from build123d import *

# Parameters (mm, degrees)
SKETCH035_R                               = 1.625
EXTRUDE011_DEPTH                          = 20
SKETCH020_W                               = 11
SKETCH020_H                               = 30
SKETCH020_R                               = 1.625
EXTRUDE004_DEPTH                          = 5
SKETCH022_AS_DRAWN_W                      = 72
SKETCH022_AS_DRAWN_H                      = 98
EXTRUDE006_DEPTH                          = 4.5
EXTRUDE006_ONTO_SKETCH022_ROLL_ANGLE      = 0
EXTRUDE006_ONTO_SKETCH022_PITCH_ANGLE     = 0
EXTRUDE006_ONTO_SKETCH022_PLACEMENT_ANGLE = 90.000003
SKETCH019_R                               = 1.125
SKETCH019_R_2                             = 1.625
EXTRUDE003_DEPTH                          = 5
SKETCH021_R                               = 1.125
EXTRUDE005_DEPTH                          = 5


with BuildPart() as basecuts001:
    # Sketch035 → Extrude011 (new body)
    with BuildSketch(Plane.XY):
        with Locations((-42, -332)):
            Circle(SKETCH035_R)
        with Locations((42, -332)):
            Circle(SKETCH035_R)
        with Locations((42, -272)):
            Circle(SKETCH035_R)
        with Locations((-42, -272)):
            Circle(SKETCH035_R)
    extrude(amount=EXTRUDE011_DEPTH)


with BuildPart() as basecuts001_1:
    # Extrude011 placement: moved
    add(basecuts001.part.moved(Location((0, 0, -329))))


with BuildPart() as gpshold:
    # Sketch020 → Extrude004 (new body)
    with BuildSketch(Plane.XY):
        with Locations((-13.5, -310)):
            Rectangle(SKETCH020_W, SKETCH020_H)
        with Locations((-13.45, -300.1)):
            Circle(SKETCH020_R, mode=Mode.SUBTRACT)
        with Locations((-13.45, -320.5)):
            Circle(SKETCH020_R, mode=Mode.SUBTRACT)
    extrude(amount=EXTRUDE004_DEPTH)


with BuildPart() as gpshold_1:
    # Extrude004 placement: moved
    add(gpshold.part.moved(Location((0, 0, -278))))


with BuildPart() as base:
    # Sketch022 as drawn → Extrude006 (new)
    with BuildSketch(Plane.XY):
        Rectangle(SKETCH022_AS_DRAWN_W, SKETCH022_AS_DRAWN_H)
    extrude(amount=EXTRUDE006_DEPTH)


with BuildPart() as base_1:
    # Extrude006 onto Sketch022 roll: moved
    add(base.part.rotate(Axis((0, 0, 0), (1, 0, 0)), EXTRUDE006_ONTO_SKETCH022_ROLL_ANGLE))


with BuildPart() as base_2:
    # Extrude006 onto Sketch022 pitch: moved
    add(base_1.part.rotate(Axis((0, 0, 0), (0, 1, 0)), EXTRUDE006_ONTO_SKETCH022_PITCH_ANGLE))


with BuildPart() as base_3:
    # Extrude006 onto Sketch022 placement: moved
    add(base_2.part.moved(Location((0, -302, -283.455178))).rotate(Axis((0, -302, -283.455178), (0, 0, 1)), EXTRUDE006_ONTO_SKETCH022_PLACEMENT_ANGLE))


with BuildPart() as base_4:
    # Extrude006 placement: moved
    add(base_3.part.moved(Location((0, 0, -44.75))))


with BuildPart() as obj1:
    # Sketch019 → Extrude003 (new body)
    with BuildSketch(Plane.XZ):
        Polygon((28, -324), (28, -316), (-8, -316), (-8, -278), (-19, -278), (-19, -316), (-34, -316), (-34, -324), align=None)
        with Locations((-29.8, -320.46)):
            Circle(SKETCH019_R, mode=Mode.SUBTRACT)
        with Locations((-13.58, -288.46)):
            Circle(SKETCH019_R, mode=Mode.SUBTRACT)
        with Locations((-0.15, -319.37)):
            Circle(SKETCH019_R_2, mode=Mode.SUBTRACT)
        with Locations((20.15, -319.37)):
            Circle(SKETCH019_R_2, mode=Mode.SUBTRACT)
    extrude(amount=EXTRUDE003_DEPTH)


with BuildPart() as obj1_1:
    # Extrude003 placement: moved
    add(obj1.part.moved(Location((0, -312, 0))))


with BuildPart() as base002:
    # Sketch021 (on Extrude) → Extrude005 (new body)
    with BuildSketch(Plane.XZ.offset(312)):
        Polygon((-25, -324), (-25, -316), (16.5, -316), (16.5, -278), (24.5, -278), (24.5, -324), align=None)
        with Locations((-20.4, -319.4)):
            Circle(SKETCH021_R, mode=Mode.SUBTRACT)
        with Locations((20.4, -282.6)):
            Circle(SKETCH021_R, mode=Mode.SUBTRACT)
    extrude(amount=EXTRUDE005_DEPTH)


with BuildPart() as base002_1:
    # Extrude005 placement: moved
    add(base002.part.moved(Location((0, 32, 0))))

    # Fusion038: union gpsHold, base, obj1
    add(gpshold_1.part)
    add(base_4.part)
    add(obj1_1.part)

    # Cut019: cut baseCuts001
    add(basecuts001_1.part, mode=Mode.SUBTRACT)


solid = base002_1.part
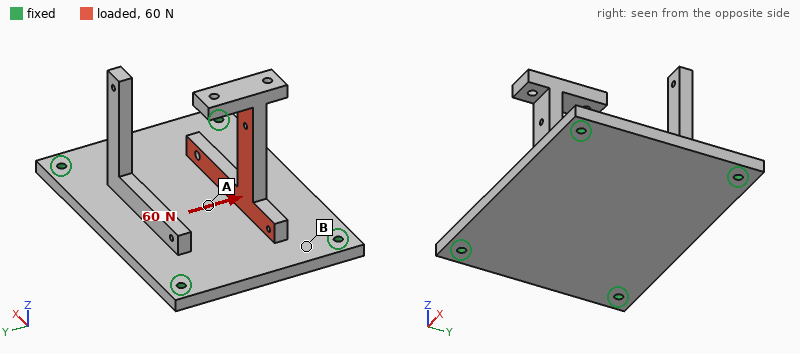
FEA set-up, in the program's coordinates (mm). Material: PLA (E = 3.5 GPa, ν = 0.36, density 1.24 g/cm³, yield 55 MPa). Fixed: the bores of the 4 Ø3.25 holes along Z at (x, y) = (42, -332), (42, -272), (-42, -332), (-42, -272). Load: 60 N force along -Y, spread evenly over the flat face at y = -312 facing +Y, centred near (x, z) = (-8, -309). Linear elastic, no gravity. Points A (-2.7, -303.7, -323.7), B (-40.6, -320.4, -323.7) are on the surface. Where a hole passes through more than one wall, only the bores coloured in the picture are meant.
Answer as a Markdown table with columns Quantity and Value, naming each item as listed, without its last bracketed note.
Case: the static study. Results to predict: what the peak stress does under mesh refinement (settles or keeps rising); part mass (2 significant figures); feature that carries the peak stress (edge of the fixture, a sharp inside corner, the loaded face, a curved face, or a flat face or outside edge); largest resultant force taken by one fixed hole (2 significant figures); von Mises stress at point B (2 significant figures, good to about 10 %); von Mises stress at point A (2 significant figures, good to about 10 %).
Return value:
| Quantity | Value |
|---|---|
| what the peak stress does under mesh refinement | keeps rising |
| part mass | 51 g |
| feature that carries the peak stress | a sharp inside corner |
| largest resultant force taken by one fixed hole | 25 N |
| von Mises stress at point B | 0.98 MPa |
| von Mises stress at point A | 1.9 MPa |
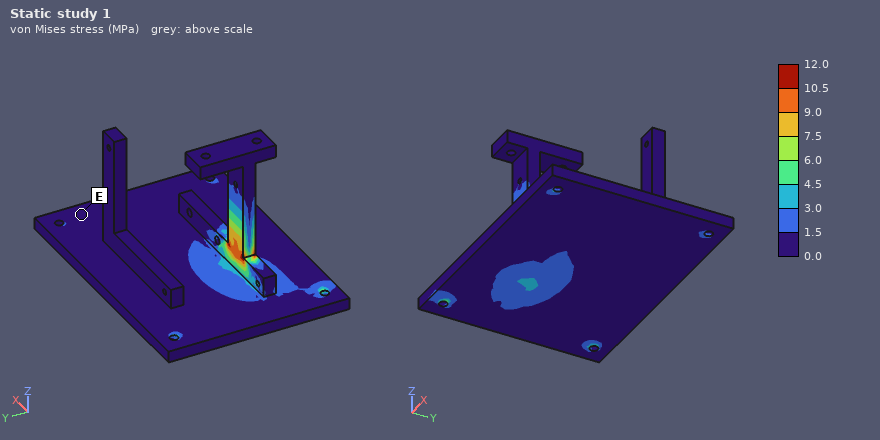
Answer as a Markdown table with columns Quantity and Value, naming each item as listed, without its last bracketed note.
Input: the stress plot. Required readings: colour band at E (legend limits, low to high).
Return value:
| Quantity | Value |
|---|---|
| colour band at E | 0.0 to 1.5 MPa |
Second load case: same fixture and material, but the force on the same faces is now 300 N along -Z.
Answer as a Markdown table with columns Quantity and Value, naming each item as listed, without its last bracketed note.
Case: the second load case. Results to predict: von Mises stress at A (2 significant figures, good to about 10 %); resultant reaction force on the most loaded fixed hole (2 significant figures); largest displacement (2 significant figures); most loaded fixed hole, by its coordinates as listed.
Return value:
| Quantity | Value |
|---|---|
| von Mises stress at A | 5.8 MPa |
| resultant reaction force on the most loaded fixed hole | 130 N |
| largest displacement | 1.4 mm |
| most loaded fixed hole, by its coordinates as listed | (-42, -332) |
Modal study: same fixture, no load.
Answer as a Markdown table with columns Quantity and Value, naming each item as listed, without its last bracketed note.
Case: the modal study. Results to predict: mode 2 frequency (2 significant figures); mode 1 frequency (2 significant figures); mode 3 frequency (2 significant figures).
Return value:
| Quantity | Value |
|---|---|
| mode 2 frequency | 630 Hz |
| mode 1 frequency | 310 Hz |
| mode 3 frequency | 680 Hz |
